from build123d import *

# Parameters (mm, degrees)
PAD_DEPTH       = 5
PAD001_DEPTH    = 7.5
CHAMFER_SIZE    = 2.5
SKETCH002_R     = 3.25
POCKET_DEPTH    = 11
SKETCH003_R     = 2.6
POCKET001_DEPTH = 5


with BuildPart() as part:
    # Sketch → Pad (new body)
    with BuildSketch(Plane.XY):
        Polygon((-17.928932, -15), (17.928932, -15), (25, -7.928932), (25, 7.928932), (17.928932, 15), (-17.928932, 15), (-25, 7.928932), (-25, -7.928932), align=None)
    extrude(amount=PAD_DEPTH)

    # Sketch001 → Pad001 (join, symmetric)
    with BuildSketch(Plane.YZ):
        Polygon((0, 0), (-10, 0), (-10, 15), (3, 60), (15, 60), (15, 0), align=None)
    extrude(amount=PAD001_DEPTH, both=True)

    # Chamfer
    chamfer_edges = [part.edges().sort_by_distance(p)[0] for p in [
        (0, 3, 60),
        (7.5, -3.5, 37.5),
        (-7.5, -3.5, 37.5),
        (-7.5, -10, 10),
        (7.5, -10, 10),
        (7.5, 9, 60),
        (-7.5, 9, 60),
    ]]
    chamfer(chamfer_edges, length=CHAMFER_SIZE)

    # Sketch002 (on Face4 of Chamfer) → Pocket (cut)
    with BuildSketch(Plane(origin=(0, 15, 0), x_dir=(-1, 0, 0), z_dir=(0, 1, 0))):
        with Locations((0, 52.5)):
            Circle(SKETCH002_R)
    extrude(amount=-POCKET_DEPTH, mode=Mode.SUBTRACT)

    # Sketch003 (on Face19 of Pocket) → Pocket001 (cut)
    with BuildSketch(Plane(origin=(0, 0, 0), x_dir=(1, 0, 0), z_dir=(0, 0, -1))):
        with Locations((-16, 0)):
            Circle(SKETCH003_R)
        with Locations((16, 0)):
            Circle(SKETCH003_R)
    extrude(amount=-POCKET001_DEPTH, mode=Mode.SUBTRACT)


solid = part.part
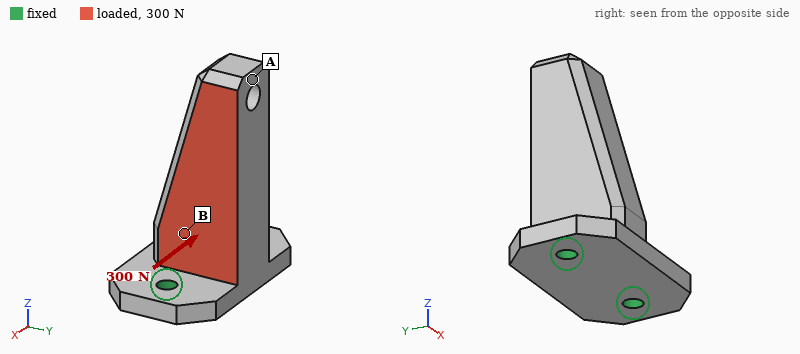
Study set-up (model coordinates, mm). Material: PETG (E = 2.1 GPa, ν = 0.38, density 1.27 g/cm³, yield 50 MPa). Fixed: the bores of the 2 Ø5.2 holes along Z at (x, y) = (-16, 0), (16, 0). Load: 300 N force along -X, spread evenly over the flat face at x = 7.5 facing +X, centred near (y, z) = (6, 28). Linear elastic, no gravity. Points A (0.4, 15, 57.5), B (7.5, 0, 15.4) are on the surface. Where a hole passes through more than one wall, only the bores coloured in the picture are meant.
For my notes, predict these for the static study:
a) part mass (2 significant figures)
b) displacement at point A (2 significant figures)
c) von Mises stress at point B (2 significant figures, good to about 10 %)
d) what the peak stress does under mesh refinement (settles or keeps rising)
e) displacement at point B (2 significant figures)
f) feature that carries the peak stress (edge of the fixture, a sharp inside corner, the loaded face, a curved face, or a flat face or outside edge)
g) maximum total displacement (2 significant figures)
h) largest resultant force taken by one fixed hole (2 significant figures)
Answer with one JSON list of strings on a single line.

["28 g", "0.90 mm", "5.3 MPa", "keeps rising", "0.18 mm", "edge of the fixture", "0.95 mm", "340 N"]
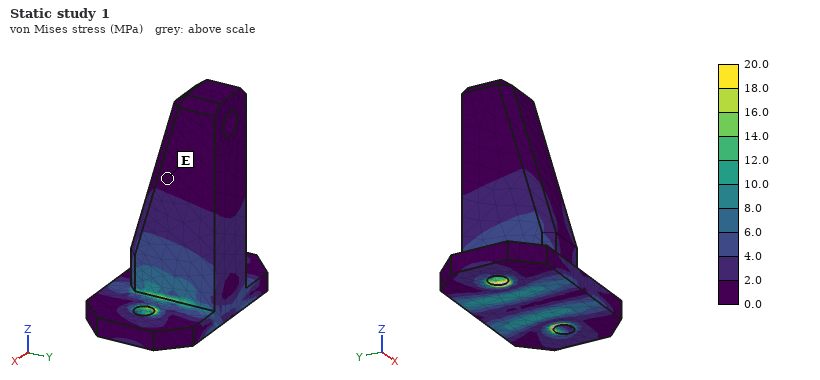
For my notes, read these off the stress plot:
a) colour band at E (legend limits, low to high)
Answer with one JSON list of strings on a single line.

["0.0 to 2.0 MPa"]
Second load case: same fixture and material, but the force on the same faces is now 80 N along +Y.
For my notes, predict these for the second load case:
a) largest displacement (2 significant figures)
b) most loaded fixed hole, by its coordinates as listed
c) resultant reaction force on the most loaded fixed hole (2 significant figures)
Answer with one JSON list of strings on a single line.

["0.60 mm", "(16, 0)", "58 N"]
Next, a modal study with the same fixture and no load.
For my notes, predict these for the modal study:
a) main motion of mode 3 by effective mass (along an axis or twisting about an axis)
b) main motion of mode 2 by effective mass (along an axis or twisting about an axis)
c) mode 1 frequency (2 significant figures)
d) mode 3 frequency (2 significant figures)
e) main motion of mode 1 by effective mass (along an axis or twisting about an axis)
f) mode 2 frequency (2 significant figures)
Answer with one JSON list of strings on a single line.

["along Z", "along X", "520 Hz", "2400 Hz", "along Y", "830 Hz"]
